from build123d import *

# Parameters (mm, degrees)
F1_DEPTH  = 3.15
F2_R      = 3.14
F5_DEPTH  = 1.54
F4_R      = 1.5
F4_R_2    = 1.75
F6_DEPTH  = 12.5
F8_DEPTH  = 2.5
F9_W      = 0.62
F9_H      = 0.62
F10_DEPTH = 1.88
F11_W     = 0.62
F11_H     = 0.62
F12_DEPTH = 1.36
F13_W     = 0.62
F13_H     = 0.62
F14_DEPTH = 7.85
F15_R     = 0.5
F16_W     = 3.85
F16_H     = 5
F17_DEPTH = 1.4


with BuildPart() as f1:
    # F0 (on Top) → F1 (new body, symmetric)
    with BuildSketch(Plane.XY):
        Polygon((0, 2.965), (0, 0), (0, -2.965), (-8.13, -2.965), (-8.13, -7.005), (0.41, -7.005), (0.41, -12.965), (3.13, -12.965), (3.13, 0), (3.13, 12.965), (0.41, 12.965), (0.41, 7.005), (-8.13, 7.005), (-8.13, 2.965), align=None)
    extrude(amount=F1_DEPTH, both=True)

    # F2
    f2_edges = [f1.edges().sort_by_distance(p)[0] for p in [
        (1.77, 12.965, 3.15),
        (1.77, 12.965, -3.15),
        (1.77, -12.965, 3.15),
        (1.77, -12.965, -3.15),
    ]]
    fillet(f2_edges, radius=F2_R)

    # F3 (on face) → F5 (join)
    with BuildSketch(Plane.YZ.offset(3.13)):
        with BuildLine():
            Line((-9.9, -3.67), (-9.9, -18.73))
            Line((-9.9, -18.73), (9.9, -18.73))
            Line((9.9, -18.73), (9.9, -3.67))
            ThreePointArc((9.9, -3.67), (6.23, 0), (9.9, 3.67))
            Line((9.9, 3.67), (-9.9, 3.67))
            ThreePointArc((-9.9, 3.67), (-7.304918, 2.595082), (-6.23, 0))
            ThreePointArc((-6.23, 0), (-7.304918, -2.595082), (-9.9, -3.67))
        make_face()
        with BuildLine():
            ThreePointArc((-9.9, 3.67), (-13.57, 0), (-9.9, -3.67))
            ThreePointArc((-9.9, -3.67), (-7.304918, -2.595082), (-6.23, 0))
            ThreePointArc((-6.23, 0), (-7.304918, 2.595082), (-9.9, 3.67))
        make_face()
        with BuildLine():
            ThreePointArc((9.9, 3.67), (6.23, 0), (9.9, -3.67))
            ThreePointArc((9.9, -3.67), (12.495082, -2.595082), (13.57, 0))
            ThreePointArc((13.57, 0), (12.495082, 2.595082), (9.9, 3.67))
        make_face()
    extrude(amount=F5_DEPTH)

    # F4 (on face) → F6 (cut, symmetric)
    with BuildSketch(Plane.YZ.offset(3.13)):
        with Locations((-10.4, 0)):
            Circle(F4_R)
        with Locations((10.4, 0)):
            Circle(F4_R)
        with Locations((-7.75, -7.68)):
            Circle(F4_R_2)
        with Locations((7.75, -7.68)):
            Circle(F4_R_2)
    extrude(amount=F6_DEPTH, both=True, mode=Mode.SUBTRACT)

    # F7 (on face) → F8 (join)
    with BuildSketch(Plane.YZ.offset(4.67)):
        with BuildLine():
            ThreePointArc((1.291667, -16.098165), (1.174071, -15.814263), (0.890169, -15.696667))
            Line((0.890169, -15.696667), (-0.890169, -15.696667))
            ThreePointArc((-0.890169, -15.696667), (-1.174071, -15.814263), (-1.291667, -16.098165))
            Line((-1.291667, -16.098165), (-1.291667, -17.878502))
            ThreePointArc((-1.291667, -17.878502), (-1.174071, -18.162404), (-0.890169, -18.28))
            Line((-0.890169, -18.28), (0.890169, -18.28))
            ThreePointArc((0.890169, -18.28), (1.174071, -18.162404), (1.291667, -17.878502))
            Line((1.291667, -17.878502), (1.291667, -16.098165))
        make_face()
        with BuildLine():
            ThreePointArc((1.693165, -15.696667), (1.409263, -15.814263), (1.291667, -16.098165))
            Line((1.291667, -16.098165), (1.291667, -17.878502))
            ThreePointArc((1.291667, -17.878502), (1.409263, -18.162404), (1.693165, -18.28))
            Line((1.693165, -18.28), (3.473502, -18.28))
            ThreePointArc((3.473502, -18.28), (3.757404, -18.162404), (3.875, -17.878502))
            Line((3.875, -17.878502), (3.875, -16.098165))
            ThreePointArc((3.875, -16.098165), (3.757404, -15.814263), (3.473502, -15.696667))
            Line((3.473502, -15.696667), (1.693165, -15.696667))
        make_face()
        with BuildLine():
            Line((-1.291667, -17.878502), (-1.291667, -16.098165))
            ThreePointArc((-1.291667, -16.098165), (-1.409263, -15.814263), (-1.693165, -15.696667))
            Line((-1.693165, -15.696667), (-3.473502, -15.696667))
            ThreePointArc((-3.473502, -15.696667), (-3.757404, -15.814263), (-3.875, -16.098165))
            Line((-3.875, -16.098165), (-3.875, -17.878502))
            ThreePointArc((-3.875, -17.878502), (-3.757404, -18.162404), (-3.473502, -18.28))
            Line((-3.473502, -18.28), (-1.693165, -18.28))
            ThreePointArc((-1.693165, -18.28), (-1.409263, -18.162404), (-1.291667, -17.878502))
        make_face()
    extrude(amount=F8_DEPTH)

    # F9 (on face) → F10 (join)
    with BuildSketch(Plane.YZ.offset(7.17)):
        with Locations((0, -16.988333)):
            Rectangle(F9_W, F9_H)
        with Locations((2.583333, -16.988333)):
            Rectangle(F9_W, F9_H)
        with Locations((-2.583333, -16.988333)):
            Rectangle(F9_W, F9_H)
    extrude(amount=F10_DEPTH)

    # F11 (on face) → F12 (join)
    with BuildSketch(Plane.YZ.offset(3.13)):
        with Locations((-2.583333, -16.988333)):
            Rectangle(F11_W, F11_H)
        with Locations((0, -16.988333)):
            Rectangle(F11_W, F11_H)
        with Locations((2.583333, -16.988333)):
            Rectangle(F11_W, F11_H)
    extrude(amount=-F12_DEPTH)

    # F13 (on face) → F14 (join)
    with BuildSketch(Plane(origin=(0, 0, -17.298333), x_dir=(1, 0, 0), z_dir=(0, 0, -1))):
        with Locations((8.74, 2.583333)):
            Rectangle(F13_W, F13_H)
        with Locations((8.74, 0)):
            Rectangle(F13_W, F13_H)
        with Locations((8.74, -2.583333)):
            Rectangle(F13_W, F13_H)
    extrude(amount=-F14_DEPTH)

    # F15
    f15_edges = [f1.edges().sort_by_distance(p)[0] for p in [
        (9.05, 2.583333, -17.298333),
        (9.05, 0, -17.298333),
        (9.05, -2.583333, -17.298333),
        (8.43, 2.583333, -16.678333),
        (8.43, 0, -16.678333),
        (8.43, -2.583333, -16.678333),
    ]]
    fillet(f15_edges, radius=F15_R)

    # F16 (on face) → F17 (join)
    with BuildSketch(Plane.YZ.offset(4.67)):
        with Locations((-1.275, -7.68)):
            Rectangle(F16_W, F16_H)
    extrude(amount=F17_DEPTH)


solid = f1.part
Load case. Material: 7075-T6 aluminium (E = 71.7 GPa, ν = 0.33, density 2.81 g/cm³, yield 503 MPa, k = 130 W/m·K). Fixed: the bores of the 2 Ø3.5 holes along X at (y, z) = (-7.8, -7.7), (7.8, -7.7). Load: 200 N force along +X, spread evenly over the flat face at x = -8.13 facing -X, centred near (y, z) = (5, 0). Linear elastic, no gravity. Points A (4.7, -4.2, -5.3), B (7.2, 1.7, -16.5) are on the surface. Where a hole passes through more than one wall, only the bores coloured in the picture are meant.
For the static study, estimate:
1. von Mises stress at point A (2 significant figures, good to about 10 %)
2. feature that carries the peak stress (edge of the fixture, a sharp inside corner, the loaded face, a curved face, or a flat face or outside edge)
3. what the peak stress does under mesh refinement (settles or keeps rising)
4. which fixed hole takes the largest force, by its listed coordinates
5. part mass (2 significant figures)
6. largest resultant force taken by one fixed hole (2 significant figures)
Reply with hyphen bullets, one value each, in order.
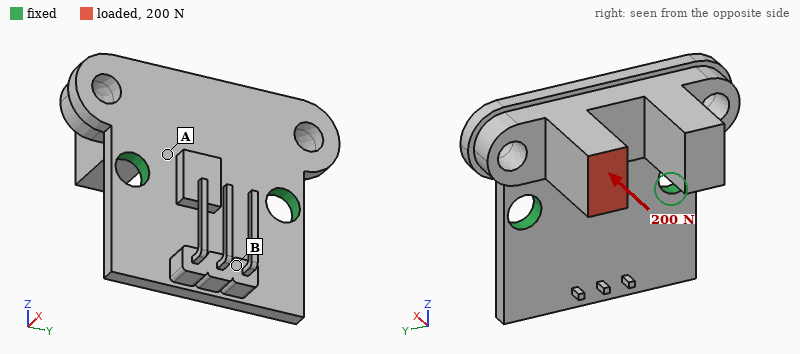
- 71 MPa
- edge of the fixture
- keeps rising
- (7.8, -7.7)
- 4.5 g
- 160 N
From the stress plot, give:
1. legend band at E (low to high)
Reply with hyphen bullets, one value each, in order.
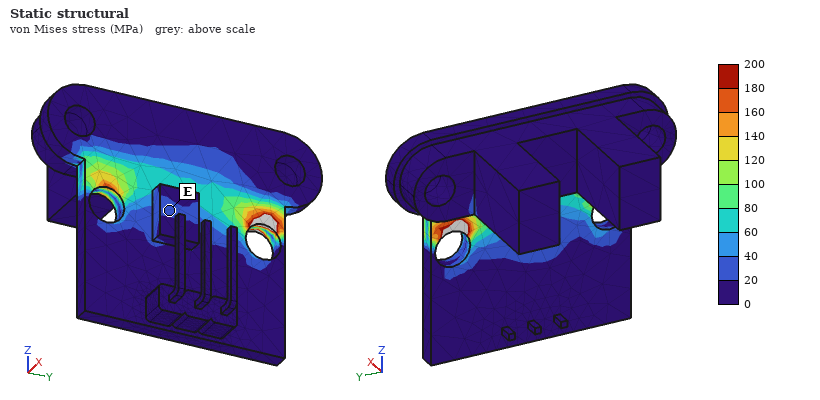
- 20 to 40 MPa
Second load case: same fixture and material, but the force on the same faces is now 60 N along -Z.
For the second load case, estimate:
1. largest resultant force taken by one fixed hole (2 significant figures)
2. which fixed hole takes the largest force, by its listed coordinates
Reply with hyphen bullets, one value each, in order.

- 50 N
- (7.8, -7.7)
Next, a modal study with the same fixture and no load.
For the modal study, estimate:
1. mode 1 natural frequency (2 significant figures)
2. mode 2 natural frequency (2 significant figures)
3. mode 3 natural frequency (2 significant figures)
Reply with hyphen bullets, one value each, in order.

- 4100 Hz
- 6300 Hz
- 6300 Hz
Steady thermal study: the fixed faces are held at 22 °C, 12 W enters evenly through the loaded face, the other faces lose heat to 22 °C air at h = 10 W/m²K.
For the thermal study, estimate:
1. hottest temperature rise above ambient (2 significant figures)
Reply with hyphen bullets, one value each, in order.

- 57 K
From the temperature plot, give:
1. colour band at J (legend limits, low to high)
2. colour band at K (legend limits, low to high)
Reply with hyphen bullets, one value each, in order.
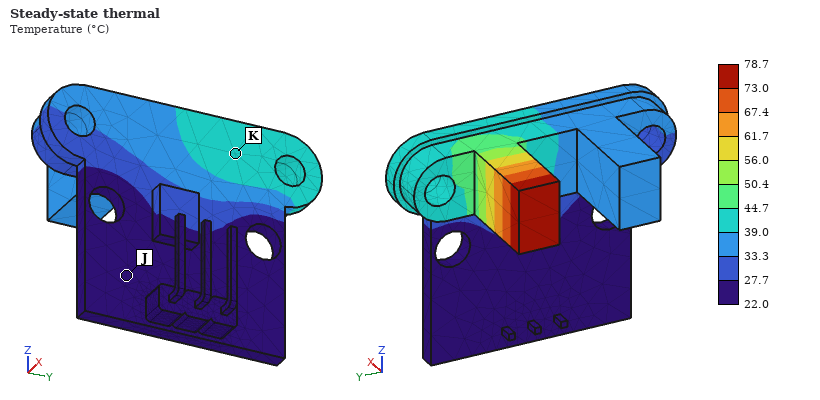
- 22.0 to 27.7 °C
- 39.0 to 44.7 °C
